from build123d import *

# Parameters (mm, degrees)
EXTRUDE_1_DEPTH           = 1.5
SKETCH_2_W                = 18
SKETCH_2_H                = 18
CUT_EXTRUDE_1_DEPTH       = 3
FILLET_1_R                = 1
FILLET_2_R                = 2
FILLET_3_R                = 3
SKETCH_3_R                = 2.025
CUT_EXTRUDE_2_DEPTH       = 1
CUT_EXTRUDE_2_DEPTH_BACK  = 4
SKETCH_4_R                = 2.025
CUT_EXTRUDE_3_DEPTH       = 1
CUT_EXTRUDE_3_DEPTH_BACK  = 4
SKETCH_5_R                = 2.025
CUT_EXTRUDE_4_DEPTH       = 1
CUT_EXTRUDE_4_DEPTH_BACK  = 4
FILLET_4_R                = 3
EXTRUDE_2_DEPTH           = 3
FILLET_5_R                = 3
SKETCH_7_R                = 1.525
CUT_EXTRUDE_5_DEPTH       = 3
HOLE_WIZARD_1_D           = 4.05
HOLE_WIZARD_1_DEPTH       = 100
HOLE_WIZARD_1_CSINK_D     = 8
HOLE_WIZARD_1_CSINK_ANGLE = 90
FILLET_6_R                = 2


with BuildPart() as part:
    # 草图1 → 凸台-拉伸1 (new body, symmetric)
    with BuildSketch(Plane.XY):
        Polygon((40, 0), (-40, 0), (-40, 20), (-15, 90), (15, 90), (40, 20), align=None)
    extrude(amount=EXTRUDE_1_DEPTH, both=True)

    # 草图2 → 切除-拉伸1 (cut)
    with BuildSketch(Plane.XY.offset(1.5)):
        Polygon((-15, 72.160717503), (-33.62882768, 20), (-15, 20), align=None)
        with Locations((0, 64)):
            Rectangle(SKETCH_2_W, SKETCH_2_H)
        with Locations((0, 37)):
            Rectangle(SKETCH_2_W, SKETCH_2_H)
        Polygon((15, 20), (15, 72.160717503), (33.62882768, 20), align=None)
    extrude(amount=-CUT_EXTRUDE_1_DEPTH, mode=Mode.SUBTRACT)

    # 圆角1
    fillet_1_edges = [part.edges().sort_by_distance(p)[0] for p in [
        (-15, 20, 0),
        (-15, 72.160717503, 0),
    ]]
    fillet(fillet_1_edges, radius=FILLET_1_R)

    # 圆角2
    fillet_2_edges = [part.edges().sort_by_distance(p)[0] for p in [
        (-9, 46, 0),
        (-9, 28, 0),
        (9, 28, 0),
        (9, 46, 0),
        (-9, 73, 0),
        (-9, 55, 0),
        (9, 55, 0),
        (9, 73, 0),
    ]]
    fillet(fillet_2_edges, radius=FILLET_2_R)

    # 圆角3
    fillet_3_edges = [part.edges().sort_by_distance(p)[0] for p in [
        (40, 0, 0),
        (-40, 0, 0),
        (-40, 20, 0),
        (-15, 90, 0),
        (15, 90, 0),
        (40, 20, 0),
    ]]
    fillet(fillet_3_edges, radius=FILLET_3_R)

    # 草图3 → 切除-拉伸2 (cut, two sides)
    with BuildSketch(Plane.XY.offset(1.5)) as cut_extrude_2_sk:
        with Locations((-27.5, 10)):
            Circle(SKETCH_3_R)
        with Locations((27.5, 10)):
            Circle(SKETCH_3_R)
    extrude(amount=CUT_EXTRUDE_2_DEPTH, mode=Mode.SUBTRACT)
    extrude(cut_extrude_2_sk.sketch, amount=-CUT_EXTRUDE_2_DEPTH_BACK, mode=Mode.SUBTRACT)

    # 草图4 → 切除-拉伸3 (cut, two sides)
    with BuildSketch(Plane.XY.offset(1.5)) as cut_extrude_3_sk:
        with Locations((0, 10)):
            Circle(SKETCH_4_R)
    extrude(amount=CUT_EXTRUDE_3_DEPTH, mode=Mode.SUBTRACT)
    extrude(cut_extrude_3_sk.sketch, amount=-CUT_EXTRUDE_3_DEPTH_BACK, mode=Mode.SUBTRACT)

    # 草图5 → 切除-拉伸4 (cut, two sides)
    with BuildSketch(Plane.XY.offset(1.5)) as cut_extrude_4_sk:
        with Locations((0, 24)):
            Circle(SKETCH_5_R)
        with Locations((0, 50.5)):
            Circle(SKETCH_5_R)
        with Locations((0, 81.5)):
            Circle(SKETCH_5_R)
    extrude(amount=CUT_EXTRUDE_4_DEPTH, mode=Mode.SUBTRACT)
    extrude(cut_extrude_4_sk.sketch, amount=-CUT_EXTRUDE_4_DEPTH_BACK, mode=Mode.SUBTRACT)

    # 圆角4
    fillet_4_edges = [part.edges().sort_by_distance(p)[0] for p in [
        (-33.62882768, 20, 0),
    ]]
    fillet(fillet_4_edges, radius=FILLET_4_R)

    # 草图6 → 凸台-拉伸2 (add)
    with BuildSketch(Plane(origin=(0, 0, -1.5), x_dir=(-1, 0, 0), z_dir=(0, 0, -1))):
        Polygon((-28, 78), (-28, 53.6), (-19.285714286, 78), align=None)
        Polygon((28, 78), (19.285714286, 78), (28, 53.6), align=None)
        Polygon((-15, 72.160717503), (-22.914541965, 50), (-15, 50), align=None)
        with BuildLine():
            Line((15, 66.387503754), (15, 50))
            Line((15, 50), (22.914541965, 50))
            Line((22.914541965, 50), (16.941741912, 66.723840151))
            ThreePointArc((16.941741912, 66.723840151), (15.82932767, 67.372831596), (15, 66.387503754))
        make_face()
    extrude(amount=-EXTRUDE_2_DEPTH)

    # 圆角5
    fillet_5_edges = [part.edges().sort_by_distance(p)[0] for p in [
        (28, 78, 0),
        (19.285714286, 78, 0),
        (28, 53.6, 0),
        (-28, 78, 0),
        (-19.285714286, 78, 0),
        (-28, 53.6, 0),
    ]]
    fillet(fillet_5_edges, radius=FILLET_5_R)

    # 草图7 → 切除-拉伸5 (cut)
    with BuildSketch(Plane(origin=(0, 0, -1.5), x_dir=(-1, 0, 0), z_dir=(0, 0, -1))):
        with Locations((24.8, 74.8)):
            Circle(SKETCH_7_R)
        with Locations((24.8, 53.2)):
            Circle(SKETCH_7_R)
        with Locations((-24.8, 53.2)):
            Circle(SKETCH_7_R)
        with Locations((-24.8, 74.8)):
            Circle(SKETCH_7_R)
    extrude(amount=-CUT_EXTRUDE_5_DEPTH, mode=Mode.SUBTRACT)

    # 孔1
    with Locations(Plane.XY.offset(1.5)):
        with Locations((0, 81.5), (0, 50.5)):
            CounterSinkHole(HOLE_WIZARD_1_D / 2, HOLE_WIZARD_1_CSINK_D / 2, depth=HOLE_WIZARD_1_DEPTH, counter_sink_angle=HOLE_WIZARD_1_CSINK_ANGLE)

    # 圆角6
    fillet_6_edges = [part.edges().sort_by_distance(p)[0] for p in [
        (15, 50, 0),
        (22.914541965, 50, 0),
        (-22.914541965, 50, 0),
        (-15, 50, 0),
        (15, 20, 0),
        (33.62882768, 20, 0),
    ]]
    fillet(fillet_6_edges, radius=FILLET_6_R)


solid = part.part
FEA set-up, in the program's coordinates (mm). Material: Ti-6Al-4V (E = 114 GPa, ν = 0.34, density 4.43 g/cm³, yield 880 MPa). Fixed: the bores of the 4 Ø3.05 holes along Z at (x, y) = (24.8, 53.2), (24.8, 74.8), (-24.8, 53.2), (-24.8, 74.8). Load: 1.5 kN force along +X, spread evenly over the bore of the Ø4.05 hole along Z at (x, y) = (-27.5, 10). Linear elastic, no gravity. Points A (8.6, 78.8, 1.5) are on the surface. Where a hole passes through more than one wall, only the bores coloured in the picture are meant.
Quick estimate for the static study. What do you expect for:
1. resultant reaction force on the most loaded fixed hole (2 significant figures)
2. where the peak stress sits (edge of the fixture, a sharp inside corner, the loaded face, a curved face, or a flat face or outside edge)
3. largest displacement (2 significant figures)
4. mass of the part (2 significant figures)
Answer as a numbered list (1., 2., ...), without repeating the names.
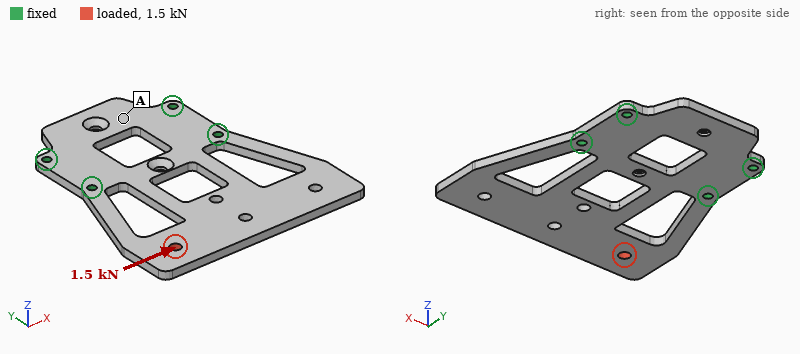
1. 1.1 kN
2. a curved face
3. 0.20 mm
4. 54 g
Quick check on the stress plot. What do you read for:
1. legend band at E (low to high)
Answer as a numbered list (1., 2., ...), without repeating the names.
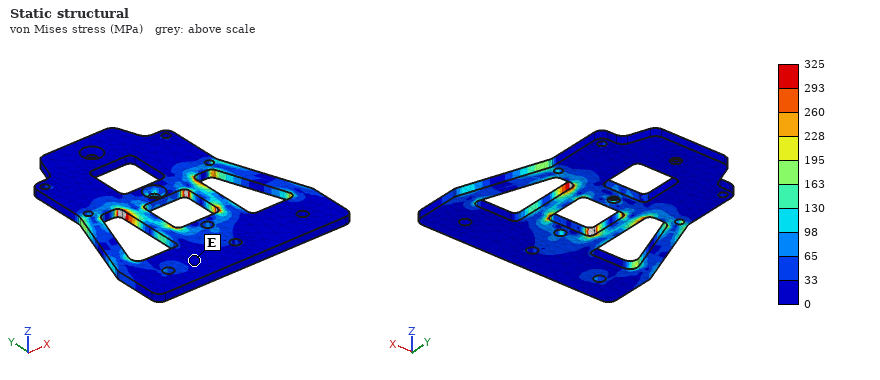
1. 0 to 33 MPa
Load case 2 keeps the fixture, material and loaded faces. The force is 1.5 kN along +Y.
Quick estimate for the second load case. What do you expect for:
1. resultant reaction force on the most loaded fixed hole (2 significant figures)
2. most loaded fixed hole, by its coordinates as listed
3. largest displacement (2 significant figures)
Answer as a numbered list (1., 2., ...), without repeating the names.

1. 1.3 kN
2. (-24.8, 53.2)
3. 56 µm
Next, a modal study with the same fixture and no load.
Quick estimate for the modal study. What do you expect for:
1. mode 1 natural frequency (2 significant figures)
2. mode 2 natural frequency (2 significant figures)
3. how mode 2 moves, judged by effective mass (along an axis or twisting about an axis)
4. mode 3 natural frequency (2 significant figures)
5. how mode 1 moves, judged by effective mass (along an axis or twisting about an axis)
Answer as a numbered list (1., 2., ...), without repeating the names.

1. 500 Hz
2. 1100 Hz
3. twisting about Y
4. 2700 Hz
5. along Z
